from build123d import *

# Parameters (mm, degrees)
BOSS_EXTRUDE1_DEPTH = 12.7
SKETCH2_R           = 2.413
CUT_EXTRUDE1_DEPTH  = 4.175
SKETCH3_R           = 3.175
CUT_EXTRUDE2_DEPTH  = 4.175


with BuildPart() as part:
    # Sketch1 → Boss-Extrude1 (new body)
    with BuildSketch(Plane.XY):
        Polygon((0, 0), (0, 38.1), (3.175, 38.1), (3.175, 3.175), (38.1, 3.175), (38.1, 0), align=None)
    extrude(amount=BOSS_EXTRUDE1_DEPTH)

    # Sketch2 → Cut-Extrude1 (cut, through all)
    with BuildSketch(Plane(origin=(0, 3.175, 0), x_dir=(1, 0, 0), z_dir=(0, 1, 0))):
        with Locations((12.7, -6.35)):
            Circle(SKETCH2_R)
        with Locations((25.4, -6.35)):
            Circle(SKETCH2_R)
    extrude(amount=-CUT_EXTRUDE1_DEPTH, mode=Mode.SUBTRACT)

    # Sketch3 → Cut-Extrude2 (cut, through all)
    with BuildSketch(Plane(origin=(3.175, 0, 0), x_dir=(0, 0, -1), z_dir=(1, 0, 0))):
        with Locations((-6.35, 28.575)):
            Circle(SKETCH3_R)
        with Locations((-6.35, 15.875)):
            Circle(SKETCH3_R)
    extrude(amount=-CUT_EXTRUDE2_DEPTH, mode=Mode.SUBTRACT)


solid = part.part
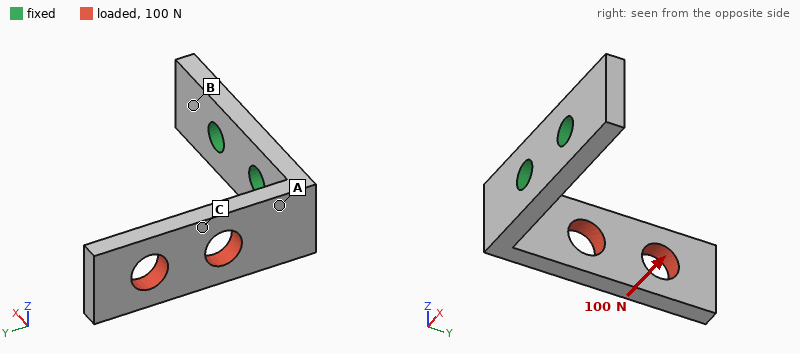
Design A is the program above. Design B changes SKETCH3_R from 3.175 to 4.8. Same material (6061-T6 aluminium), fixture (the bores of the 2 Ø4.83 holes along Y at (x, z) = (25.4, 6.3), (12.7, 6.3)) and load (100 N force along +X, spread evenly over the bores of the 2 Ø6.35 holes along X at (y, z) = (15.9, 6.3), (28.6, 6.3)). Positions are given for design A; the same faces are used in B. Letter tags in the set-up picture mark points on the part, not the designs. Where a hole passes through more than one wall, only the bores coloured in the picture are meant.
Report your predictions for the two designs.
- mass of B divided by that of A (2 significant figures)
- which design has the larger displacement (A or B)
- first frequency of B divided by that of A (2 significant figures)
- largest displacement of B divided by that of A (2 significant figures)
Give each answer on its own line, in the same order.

0.90
B
1.0
1.2
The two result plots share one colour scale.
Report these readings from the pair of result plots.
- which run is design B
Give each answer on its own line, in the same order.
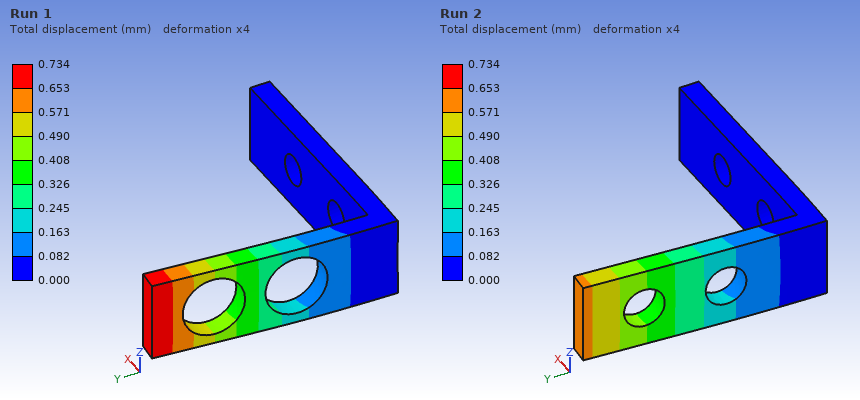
Run 1
